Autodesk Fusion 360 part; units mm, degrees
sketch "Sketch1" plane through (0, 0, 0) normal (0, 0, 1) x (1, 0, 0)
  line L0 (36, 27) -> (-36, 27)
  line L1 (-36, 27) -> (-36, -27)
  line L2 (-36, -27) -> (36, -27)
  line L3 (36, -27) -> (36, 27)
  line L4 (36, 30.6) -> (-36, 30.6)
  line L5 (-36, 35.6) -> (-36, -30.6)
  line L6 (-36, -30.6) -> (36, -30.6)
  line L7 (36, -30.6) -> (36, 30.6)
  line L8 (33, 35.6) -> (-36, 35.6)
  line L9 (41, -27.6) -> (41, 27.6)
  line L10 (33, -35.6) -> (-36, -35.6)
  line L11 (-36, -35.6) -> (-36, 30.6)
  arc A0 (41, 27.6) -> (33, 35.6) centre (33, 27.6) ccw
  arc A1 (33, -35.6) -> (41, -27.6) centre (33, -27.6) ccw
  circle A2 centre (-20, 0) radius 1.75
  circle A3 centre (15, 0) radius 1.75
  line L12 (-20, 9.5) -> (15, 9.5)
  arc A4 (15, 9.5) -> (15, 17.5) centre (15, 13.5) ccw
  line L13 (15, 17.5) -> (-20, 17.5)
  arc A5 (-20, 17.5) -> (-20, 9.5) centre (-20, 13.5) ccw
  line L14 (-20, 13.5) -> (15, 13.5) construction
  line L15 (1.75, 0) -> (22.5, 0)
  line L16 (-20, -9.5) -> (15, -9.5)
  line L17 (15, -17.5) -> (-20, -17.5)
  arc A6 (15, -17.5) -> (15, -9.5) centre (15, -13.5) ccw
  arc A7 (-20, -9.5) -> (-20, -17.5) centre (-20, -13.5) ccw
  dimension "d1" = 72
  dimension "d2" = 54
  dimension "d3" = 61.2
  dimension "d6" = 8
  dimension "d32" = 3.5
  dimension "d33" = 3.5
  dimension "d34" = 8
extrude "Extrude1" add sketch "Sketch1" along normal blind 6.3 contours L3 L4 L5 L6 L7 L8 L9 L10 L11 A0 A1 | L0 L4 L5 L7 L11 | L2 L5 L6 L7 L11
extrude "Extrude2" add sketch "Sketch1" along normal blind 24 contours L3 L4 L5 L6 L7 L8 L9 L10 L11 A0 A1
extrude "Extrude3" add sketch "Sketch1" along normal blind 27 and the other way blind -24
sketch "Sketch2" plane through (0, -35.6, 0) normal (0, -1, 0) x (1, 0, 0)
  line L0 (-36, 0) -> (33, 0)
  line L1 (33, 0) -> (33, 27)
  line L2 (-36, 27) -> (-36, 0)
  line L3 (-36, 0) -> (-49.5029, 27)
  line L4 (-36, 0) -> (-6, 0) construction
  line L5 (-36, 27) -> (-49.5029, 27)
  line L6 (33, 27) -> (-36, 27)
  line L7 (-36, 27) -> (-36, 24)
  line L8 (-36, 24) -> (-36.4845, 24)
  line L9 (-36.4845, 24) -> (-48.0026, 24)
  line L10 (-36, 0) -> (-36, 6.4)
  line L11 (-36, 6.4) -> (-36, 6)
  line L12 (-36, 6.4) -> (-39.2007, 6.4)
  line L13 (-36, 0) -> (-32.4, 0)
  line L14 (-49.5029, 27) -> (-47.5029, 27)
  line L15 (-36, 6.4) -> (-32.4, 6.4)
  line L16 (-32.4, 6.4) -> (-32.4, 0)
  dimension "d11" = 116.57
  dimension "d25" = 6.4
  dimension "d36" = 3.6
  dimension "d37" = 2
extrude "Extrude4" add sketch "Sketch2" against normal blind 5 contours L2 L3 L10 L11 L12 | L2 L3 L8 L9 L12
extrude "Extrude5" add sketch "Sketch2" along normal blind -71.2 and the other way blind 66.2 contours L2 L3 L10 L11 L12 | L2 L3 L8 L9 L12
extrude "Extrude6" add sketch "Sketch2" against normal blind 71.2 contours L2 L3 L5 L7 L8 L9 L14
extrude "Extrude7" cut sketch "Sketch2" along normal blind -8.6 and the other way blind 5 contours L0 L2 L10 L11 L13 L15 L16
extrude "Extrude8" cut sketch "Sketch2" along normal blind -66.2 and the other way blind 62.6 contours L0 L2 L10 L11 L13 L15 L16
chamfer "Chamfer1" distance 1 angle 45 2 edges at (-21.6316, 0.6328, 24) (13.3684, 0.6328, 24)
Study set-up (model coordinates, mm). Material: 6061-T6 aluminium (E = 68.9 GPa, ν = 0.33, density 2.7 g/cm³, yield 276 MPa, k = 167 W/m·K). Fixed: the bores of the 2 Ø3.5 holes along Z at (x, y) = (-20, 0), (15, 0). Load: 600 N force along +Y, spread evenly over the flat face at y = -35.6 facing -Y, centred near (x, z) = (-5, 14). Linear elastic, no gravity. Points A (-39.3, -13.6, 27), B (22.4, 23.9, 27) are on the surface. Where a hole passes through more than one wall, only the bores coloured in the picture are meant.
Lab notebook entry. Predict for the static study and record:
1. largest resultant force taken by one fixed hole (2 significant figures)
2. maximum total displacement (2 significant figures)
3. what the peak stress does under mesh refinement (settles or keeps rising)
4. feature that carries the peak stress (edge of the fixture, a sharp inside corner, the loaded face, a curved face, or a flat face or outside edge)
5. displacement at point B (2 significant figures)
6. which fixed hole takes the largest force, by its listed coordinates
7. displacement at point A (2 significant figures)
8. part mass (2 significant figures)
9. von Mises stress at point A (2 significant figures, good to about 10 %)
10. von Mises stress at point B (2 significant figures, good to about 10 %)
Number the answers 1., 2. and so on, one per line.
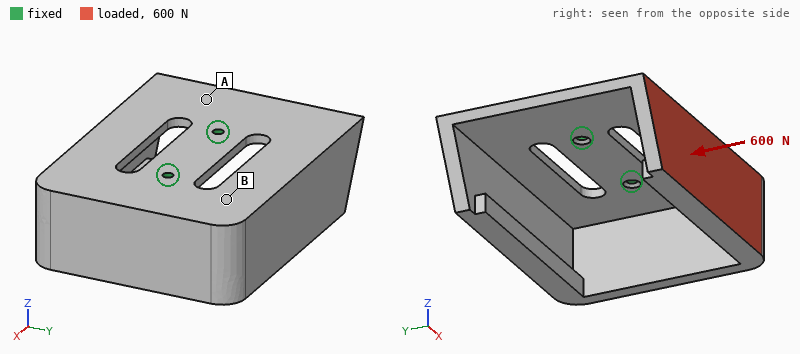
1. 350 N
2. 0.57 mm
3. keeps rising
4. edge of the fixture
5. 0.26 mm
6. (-20, 0)
7. 0.10 mm
8. 130 g
9. 34 MPa
10. 11 MPa
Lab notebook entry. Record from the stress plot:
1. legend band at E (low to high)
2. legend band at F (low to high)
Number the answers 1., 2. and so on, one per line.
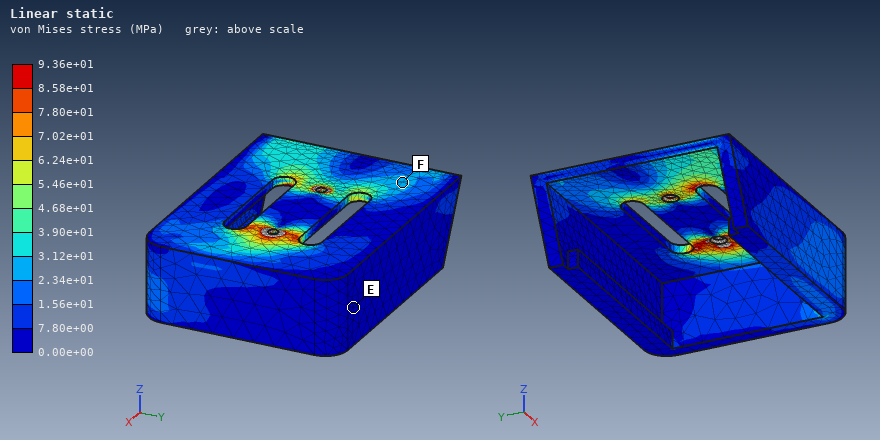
1. 0.00e+00 to 7.80e+00 MPa
2. 2.34e+01 to 3.12e+01 MPa
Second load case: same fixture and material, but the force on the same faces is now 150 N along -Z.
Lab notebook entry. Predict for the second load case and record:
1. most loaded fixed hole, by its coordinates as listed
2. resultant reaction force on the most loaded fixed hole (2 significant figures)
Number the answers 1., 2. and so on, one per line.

1. (-20, 0)
2. 92 N
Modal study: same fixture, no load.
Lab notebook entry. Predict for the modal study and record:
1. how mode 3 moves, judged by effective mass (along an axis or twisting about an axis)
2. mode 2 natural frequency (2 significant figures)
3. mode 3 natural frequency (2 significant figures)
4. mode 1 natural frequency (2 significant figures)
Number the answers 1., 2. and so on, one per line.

1. along Z
2. 950 Hz
3. 1200 Hz
4. 410 Hz
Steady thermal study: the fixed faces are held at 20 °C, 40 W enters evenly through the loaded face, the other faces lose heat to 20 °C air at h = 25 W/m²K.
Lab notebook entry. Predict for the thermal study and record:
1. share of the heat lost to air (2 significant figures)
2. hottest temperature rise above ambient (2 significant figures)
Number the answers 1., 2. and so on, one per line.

1. 32 %
2. 50 K
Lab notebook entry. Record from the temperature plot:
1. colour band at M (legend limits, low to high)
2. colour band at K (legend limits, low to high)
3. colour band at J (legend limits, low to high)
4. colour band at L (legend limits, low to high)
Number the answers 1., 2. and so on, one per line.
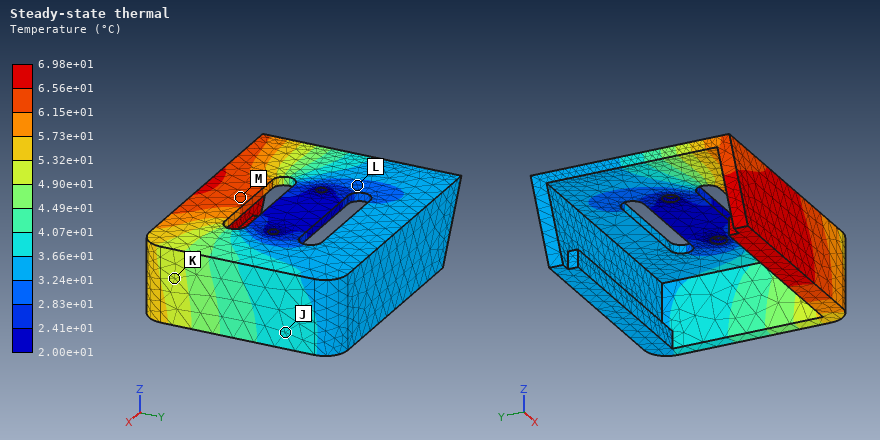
1. 6.15e+01 to 6.56e+01 °C
2. 4.90e+01 to 5.32e+01 °C
3. 3.66e+01 to 4.07e+01 °C
4. 2.83e+01 to 3.24e+01 °C
